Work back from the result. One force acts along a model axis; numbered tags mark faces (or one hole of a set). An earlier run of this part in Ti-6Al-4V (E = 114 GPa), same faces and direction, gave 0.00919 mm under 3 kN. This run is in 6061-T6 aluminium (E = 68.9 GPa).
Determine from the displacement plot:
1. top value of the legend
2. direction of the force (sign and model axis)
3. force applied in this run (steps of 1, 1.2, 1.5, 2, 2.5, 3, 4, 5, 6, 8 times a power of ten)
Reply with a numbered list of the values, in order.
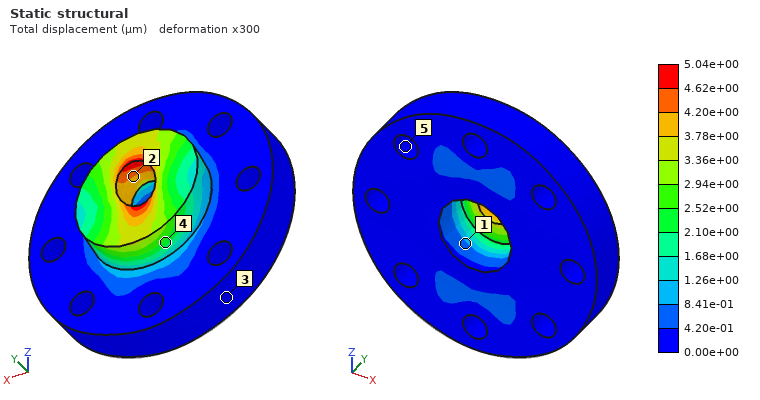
1. 5.04e+00 µm
2. +Z
3. 1 kN
